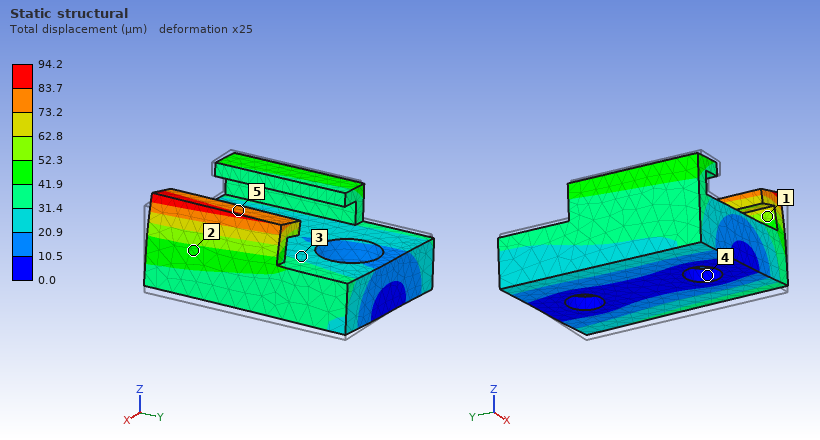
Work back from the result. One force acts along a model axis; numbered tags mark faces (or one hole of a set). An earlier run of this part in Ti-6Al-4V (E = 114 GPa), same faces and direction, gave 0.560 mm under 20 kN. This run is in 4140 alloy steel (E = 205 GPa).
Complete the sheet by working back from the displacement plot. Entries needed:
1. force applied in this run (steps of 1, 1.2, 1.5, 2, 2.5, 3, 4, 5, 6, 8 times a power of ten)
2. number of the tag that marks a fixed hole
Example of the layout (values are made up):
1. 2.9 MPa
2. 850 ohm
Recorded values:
1. 6 kN
2. 4
